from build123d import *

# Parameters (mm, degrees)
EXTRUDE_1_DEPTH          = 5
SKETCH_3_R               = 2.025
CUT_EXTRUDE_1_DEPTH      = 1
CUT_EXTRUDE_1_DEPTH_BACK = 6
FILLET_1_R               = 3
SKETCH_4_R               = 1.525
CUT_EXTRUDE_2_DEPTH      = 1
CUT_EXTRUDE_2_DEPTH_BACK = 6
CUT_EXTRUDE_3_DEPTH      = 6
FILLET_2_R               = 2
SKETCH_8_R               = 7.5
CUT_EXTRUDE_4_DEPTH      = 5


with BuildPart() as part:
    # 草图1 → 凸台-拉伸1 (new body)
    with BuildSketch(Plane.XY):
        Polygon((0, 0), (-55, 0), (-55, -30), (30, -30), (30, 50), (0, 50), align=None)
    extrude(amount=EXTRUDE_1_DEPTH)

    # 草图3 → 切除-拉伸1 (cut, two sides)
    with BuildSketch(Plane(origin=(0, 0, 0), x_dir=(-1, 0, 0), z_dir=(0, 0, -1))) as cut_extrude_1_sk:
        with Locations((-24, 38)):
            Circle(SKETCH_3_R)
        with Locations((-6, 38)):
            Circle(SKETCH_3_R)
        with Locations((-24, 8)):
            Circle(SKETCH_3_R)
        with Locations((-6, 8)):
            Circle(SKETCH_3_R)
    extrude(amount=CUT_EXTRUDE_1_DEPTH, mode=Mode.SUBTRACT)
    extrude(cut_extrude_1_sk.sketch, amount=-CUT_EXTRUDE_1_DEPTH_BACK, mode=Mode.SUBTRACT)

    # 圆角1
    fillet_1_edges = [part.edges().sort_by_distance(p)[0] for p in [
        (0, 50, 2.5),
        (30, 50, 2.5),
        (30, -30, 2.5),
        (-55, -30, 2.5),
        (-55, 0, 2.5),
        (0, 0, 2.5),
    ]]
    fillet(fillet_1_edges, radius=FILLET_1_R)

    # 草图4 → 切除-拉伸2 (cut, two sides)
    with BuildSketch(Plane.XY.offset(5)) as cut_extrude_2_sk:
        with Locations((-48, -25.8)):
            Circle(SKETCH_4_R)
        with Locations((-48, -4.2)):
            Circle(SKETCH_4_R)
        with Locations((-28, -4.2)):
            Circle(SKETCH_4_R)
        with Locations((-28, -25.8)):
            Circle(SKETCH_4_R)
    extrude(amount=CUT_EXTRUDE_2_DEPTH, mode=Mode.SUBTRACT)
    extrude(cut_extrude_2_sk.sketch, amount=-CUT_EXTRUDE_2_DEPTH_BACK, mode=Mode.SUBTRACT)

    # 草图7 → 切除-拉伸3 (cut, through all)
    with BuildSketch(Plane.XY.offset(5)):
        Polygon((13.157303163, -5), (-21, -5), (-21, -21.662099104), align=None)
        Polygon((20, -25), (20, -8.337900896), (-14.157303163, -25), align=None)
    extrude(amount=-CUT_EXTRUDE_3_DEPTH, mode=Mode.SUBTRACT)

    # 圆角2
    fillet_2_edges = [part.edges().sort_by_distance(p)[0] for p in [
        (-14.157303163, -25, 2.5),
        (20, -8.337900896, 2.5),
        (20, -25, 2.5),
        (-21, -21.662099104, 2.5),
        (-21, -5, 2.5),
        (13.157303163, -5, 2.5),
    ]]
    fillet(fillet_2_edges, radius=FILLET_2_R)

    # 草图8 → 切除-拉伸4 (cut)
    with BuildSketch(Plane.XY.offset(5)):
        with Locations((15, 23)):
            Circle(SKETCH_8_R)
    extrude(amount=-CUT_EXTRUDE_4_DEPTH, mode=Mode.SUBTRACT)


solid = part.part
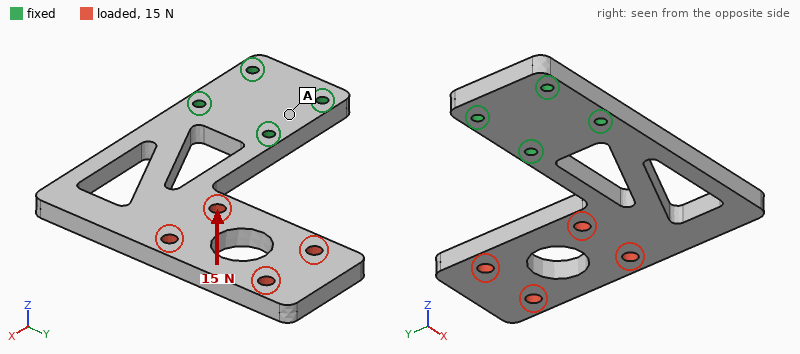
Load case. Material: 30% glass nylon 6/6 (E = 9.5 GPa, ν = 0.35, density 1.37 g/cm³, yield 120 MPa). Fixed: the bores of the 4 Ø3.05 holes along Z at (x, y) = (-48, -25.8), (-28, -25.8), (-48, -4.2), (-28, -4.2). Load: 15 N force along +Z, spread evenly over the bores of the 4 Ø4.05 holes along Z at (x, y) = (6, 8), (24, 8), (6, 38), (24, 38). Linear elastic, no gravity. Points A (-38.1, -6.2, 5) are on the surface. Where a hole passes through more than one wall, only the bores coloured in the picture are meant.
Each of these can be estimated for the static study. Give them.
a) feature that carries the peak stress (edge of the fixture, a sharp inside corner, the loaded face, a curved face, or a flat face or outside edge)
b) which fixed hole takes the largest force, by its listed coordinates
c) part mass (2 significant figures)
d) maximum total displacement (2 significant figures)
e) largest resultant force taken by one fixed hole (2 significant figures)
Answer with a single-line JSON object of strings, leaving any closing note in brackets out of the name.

{"feature that carries the peak stress": "a curved face", "which fixed hole takes the largest force, by its listed coordinates": "(-28, -4.2)", "part mass": "22 g", "maximum total displacement": "1.1 mm", "largest resultant force taken by one fixed hole": "31 N"}
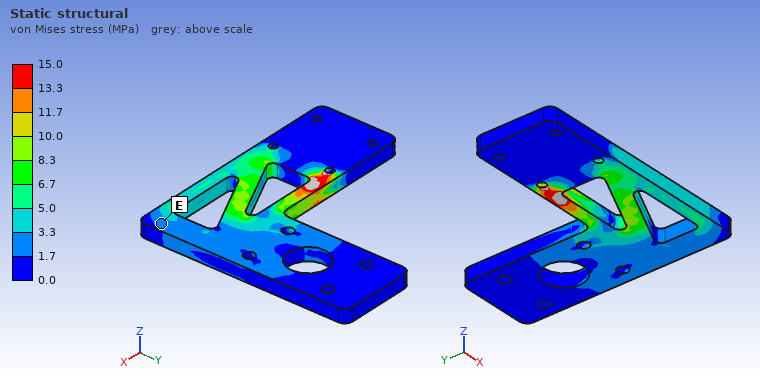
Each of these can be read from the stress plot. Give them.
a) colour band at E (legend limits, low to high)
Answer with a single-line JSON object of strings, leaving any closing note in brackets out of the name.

{"colour band at E": "1.7 to 3.3 MPa"}
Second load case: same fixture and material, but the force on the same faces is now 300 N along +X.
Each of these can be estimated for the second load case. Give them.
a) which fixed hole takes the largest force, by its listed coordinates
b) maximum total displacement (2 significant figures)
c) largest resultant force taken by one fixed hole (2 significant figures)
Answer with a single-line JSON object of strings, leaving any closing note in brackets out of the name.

{"which fixed hole takes the largest force, by its listed coordinates": "(-28, -4.2)", "maximum total displacement": "0.77 mm", "largest resultant force taken by one fixed hole": "600 N"}
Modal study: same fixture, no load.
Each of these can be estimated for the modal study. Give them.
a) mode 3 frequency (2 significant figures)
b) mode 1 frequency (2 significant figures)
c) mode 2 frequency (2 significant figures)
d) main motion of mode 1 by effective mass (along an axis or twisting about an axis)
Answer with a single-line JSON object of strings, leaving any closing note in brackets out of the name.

{"mode 3 frequency": "1100 Hz", "mode 1 frequency": "230 Hz", "mode 2 frequency": "540 Hz", "main motion of mode 1 by effective mass": "along Z"}
